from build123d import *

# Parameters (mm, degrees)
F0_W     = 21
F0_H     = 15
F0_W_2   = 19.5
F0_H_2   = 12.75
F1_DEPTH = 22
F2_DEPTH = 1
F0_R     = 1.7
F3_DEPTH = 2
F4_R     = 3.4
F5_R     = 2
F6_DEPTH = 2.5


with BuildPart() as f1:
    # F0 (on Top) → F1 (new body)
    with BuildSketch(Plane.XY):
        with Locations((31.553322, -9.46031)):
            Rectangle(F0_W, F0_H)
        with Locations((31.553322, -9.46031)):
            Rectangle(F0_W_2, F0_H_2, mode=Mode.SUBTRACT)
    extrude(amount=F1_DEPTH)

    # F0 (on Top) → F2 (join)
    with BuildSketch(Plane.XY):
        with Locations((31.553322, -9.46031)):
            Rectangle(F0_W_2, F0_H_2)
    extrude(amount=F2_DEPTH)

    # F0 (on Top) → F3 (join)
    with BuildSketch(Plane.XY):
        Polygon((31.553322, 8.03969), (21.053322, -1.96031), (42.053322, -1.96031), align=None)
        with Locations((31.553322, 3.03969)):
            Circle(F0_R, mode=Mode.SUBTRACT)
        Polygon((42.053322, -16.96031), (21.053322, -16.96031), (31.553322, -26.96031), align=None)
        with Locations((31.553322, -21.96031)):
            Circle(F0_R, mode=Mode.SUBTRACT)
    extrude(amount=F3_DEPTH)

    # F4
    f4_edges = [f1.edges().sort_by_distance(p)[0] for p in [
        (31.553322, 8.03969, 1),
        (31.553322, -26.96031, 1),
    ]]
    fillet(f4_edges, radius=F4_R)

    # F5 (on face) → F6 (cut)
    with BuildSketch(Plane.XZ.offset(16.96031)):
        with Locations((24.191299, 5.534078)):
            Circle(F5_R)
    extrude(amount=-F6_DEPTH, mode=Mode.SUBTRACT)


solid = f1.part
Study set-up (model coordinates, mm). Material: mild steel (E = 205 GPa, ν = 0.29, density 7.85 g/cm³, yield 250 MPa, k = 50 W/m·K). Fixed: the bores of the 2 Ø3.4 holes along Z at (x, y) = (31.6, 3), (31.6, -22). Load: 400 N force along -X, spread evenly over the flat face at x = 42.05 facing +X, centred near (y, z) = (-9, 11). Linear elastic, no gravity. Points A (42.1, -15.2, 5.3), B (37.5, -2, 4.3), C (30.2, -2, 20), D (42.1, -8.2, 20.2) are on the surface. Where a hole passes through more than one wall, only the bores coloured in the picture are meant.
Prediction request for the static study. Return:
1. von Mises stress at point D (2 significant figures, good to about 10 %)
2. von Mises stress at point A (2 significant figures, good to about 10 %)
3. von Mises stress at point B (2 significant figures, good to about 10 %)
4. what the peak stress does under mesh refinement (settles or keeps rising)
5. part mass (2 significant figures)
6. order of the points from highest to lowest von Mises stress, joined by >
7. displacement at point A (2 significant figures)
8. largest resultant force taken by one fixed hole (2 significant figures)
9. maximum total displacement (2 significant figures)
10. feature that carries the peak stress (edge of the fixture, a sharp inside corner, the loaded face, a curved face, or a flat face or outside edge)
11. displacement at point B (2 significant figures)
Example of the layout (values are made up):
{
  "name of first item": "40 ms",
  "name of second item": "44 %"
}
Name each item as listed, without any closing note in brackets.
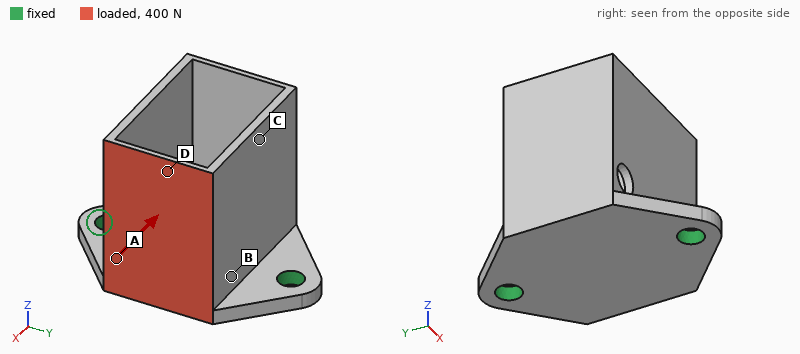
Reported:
{
  "von Mises stress at point D": "120 MPa",
  "von Mises stress at point A": "67 MPa",
  "von Mises stress at point B": "34 MPa",
  "what the peak stress does under mesh refinement": "keeps rising",
  "part mass": "16 g",
  "order of the points from highest to lowest von Mises stress, joined by >": "D > A > B > C",
  "displacement at point A": "33 µm",
  "largest resultant force taken by one fixed hole": "200 N",
  "maximum total displacement": "93 µm",
  "feature that carries the peak stress": "edge of the fixture",
  "displacement at point B": "19 µm"
}
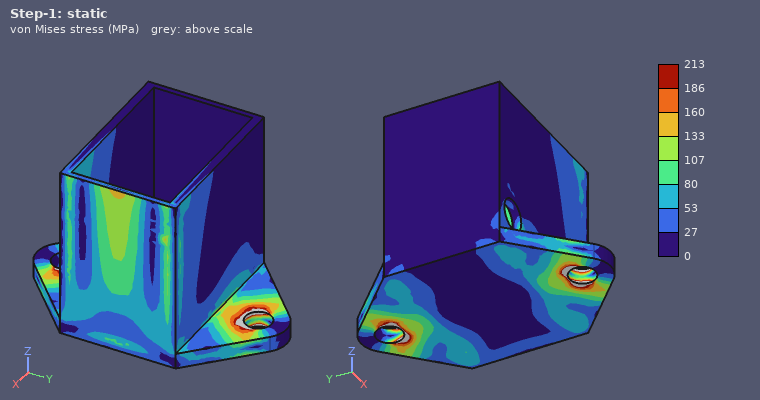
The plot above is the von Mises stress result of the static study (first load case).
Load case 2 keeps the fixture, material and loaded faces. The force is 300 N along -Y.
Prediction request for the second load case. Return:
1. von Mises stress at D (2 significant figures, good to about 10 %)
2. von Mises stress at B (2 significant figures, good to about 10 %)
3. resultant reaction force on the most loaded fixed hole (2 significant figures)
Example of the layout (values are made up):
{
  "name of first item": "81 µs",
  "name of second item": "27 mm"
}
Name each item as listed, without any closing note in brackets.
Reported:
{
  "von Mises stress at D": "21 MPa",
  "von Mises stress at B": "54 MPa",
  "resultant reaction force on the most loaded fixed hole": "250 N"
}
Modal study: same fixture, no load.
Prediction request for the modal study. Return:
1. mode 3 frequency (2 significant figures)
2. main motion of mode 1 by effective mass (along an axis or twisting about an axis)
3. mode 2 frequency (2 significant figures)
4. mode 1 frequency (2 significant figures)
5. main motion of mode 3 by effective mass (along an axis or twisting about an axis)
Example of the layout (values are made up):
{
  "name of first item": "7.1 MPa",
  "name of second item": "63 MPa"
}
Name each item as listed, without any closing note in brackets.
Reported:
{
  "mode 3 frequency": "7700 Hz",
  "main motion of mode 1 by effective mass": "along X",
  "mode 2 frequency": "6600 Hz",
  "mode 1 frequency": "3900 Hz",
  "main motion of mode 3 by effective mass": "along Y"
}
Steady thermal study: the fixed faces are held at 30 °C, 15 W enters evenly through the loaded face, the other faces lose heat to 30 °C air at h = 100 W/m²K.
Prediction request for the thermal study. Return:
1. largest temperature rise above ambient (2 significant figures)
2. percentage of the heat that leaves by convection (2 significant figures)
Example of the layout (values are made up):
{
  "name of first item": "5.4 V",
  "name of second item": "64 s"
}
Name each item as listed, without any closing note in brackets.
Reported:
{
  "largest temperature rise above ambient": "80 K",
  "percentage of the heat that leaves by convection": "57 %"
}
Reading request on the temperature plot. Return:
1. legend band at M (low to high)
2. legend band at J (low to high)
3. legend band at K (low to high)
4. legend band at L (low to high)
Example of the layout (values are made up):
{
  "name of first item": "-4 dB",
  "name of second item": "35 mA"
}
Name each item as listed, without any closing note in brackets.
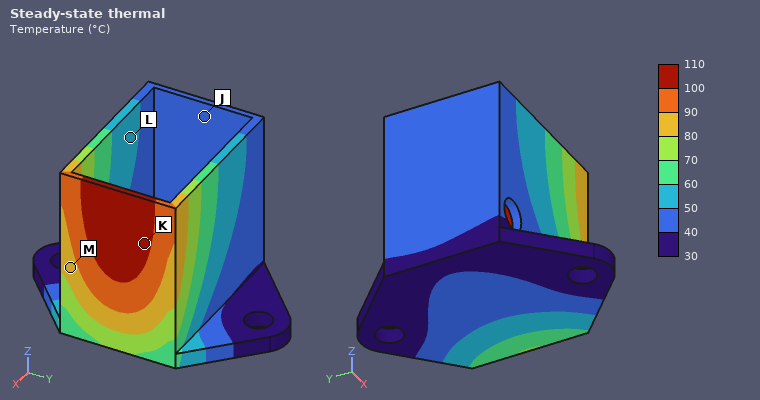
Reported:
{
  "legend band at M": "80 to 90 °C",
  "legend band at J": "40 to 50 °C",
  "legend band at K": "100 to 110 °C",
  "legend band at L": "50 to 60 °C"
}
